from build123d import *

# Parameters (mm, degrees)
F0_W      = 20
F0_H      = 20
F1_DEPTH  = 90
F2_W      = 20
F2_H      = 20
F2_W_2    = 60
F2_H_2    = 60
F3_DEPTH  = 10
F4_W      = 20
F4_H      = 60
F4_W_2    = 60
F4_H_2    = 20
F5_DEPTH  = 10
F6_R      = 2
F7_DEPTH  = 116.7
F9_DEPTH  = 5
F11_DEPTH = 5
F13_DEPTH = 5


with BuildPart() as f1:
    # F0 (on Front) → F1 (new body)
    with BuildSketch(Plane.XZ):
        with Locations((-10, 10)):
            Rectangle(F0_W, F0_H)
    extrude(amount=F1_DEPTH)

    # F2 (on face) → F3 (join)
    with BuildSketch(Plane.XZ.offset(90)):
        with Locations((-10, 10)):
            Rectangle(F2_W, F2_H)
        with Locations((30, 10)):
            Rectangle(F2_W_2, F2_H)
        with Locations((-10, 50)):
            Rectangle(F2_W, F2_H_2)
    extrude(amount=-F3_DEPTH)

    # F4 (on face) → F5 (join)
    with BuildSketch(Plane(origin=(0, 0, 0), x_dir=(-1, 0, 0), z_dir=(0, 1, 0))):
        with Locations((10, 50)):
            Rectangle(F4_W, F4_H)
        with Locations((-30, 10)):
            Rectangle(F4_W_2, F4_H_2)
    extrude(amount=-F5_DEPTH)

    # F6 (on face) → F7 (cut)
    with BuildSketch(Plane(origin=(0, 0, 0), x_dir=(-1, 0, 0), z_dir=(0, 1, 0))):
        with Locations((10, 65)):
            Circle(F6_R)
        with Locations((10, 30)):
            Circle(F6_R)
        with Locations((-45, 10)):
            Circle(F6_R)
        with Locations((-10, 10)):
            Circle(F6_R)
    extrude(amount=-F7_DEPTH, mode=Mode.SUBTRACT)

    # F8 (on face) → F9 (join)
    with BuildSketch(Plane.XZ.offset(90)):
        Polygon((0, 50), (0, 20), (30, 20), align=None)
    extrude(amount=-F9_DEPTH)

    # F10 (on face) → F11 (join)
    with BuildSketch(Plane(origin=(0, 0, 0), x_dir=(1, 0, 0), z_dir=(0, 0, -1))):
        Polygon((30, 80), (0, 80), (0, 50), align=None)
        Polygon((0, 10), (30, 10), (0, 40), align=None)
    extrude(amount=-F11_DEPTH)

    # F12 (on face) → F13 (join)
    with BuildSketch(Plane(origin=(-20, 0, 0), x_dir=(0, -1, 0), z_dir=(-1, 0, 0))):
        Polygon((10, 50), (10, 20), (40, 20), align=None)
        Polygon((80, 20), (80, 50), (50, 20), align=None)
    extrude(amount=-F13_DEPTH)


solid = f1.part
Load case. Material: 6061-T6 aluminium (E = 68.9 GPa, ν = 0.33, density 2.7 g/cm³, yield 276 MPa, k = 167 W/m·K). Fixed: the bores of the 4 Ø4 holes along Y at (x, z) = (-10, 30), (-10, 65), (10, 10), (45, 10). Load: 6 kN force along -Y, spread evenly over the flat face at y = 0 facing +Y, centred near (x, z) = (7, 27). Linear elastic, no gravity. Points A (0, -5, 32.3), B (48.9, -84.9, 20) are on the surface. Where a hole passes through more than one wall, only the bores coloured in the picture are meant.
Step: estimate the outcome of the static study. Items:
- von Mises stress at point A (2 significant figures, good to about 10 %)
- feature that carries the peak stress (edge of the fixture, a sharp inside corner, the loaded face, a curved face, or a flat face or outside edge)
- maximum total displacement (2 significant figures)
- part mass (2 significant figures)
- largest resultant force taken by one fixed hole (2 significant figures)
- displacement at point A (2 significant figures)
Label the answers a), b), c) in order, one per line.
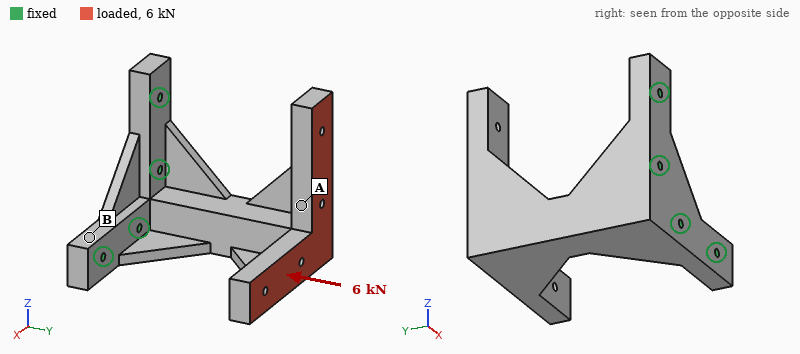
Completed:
a) 40 MPa
b) a flat face or outside edge
c) 1.2 mm
d) 250 g
e) 2.2 kN
f) 0.64 mm
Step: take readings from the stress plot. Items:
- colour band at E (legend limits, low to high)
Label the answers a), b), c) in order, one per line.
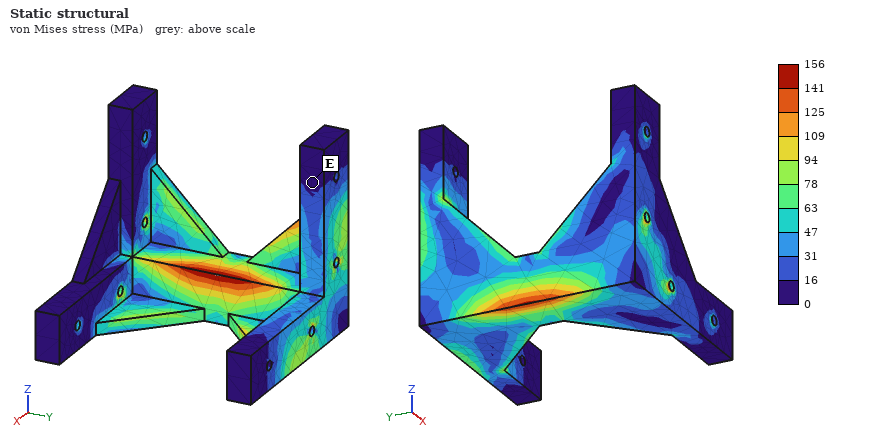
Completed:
a) 0 to 16 MPa
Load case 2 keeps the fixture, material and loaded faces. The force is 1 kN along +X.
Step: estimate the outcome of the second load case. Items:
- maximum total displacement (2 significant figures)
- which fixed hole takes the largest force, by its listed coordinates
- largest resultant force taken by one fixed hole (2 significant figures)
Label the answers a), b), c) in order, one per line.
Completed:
a) 0.50 mm
b) (-10, 30)
c) 2.1 kN
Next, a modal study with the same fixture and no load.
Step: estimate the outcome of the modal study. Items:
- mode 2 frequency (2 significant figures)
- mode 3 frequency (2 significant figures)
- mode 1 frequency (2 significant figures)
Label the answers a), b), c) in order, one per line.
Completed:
a) 1000 Hz
b) 1800 Hz
c) 810 Hz
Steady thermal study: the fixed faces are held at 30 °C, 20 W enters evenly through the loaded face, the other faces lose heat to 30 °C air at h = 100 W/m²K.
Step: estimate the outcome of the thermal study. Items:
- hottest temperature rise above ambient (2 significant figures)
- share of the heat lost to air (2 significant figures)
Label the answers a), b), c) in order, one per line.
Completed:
a) 14 K
b) 61 %
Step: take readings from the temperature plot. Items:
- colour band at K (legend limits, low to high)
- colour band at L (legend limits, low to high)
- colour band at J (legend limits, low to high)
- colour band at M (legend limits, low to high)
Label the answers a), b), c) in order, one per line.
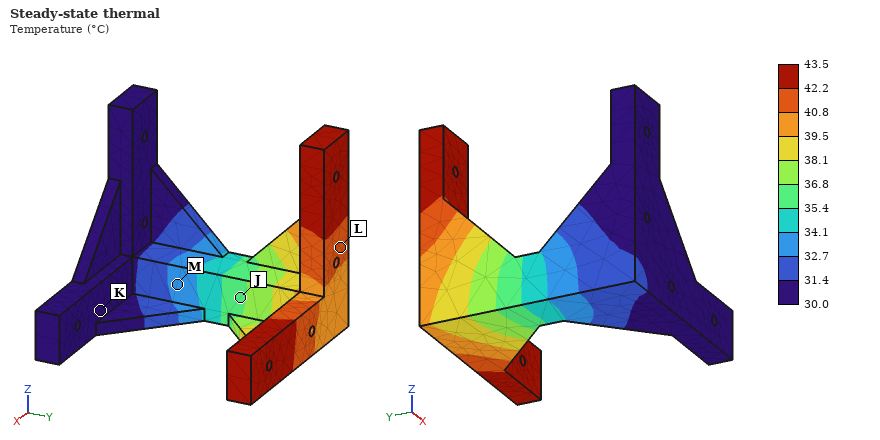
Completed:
a) 30.0 to 31.4 °C
b) 40.8 to 42.2 °C
c) 35.4 to 36.8 °C
d) 32.7 to 34.1 °C
